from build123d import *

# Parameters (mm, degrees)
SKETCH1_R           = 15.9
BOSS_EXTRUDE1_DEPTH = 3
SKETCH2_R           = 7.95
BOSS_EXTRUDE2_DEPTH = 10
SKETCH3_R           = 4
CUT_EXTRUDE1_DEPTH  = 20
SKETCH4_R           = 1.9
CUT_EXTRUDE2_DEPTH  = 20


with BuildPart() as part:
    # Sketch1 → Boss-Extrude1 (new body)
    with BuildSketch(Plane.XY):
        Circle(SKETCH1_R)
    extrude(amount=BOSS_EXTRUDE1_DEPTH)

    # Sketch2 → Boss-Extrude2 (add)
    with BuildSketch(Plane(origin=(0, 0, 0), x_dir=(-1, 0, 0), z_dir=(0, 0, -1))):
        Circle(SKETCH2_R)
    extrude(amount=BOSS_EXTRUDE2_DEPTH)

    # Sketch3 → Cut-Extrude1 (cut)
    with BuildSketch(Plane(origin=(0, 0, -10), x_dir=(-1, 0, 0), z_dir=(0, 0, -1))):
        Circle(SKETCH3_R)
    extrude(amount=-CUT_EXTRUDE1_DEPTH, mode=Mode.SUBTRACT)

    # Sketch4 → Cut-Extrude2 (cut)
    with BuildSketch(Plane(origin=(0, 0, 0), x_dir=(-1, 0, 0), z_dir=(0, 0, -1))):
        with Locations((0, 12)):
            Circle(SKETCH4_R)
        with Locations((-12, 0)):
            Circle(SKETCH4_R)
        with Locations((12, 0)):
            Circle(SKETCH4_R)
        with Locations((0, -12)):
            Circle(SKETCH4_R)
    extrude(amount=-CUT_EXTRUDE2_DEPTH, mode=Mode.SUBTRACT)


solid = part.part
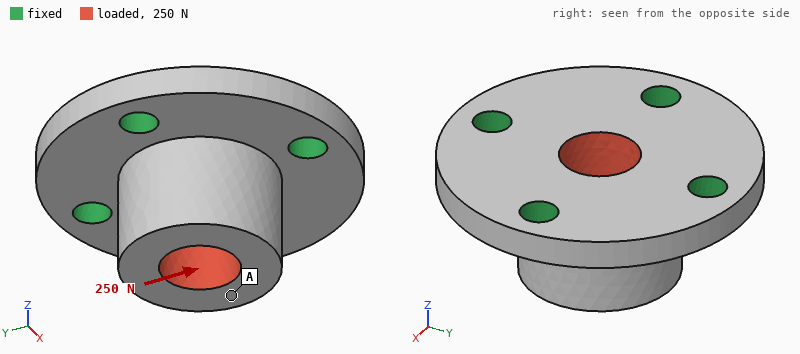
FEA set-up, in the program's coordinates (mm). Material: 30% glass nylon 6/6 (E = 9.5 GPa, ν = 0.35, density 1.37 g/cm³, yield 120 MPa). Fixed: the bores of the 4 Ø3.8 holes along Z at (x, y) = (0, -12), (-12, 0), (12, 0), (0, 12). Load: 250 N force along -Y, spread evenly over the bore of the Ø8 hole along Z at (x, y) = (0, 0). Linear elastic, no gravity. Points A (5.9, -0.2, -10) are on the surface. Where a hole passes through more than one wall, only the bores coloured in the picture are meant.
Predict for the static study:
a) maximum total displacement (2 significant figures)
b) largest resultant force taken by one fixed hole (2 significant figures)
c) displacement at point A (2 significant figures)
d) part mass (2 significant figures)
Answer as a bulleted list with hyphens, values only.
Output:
- 12 µm
- 100 N
- 9.9 µm
- 4.9 g
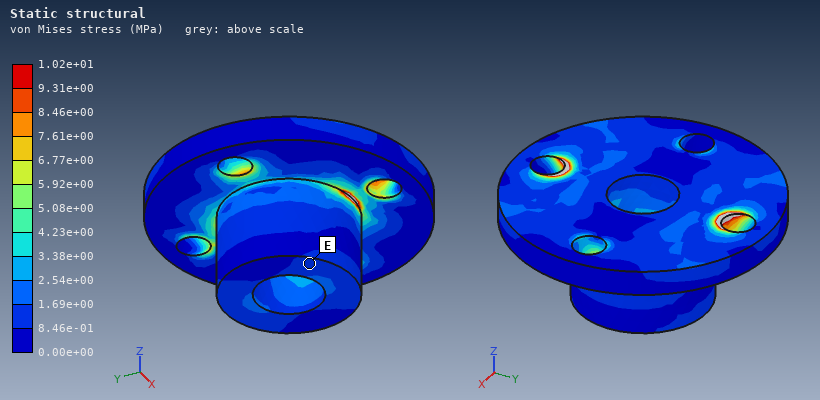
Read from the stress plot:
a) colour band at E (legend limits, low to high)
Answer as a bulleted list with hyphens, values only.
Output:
- 8.46e-01 to 1.69e+00 MPa
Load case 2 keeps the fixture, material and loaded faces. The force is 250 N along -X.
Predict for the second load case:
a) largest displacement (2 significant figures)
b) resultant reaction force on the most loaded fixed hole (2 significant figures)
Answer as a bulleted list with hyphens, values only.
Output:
- 12 µm
- 100 N
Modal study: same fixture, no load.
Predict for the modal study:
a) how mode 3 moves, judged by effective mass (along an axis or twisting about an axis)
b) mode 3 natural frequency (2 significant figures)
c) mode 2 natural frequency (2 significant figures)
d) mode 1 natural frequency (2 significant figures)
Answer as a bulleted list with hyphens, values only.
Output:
- along Z
- 19 kHz
- 16 kHz
- 16 kHz
